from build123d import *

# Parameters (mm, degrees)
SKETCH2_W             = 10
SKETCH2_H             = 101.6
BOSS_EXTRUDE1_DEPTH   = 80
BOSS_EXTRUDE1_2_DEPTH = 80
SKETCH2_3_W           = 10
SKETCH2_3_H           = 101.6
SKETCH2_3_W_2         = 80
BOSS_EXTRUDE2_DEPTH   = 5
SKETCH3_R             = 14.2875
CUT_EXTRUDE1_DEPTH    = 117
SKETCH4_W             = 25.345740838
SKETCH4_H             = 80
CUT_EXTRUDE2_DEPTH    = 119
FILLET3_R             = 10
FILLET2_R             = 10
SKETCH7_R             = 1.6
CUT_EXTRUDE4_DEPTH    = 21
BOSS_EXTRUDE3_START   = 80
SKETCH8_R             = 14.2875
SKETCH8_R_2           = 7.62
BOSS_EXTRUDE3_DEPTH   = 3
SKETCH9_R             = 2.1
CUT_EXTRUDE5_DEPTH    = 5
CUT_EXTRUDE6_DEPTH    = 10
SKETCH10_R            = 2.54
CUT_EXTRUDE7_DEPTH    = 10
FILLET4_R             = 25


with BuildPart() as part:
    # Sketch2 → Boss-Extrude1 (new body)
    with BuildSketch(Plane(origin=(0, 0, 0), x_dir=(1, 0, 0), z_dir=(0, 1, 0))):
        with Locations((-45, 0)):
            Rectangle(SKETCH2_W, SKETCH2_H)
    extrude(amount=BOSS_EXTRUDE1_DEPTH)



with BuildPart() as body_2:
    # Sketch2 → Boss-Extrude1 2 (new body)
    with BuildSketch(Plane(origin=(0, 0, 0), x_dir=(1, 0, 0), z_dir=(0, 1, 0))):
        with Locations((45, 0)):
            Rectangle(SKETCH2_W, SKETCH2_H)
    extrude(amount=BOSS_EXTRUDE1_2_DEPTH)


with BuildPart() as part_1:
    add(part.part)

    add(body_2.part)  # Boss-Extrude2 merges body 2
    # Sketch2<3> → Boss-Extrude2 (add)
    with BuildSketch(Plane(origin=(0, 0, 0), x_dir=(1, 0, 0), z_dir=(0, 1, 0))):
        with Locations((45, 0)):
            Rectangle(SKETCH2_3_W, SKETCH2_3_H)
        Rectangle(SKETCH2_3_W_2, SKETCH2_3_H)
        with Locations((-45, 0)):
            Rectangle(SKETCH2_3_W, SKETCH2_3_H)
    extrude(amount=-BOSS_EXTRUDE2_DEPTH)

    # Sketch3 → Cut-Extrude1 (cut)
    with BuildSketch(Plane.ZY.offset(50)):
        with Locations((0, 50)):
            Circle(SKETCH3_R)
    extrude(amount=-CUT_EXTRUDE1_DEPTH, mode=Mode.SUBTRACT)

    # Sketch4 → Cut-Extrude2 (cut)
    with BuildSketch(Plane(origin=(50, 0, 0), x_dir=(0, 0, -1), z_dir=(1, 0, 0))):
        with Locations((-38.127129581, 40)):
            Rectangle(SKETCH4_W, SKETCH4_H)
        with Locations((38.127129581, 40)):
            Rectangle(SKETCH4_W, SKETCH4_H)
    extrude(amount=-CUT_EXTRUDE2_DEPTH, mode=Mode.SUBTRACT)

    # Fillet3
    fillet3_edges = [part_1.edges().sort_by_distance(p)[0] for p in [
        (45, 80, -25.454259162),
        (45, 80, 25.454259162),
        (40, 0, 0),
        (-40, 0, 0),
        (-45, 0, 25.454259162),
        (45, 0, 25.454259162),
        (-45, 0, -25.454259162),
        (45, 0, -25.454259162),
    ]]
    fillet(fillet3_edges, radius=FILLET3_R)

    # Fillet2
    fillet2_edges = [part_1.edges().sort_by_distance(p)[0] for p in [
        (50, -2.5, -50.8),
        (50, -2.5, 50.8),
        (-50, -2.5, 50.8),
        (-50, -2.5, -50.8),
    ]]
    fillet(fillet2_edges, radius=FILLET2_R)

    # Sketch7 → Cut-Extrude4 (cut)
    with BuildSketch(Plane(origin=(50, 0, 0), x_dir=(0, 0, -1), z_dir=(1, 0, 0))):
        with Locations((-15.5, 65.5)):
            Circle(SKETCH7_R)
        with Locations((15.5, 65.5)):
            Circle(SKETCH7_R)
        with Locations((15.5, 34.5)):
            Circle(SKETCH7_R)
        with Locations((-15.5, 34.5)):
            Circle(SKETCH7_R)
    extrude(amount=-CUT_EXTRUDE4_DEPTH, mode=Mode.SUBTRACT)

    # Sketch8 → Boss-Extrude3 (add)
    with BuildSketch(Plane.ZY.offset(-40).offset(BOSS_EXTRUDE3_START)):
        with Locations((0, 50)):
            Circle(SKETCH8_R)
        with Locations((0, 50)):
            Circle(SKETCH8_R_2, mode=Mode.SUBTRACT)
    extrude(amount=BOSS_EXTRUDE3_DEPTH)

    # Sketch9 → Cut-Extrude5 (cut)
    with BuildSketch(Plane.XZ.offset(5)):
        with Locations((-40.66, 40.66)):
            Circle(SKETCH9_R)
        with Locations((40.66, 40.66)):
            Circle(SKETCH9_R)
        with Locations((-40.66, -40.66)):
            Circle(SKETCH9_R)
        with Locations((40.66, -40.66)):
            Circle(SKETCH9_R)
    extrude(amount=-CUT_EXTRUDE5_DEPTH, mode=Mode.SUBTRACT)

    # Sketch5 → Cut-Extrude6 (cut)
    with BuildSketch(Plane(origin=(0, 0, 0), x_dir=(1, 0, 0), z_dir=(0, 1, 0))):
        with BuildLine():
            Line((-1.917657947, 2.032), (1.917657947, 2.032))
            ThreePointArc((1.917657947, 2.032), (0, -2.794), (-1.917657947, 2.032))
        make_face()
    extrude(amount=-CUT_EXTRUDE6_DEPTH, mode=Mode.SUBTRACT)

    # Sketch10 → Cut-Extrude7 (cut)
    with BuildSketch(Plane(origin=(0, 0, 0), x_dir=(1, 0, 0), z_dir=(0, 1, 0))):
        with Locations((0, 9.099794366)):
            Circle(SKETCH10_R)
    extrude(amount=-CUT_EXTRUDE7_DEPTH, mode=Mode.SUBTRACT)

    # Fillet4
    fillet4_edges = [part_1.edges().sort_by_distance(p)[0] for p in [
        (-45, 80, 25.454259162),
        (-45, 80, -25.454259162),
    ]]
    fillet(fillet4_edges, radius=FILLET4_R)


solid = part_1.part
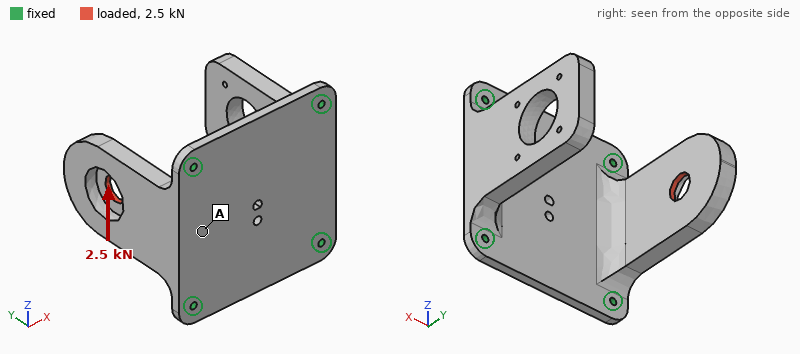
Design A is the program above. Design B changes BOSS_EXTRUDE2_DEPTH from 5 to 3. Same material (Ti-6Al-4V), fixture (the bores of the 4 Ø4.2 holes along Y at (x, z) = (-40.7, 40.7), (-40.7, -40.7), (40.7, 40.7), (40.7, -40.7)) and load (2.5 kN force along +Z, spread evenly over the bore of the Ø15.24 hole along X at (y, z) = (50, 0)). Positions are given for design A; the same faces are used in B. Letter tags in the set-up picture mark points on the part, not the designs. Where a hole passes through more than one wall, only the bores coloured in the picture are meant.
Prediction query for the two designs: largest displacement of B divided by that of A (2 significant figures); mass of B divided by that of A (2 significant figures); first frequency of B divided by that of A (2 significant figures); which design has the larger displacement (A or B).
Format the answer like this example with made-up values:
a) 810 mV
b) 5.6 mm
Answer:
a) 1.8
b) 0.83
c) 0.61
d) B
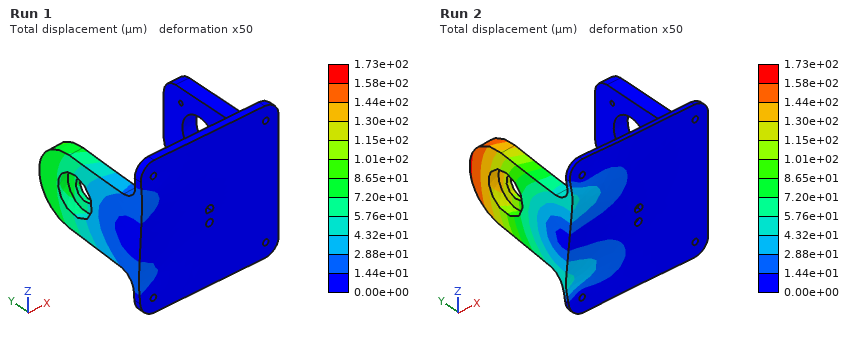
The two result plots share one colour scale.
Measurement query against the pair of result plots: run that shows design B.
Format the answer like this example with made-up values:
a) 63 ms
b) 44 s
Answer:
a) Run 2
